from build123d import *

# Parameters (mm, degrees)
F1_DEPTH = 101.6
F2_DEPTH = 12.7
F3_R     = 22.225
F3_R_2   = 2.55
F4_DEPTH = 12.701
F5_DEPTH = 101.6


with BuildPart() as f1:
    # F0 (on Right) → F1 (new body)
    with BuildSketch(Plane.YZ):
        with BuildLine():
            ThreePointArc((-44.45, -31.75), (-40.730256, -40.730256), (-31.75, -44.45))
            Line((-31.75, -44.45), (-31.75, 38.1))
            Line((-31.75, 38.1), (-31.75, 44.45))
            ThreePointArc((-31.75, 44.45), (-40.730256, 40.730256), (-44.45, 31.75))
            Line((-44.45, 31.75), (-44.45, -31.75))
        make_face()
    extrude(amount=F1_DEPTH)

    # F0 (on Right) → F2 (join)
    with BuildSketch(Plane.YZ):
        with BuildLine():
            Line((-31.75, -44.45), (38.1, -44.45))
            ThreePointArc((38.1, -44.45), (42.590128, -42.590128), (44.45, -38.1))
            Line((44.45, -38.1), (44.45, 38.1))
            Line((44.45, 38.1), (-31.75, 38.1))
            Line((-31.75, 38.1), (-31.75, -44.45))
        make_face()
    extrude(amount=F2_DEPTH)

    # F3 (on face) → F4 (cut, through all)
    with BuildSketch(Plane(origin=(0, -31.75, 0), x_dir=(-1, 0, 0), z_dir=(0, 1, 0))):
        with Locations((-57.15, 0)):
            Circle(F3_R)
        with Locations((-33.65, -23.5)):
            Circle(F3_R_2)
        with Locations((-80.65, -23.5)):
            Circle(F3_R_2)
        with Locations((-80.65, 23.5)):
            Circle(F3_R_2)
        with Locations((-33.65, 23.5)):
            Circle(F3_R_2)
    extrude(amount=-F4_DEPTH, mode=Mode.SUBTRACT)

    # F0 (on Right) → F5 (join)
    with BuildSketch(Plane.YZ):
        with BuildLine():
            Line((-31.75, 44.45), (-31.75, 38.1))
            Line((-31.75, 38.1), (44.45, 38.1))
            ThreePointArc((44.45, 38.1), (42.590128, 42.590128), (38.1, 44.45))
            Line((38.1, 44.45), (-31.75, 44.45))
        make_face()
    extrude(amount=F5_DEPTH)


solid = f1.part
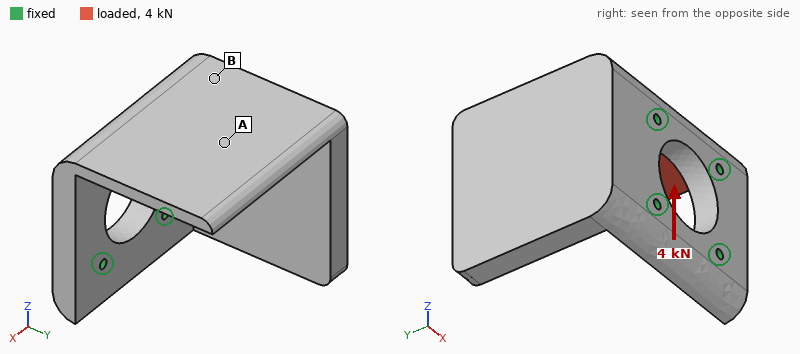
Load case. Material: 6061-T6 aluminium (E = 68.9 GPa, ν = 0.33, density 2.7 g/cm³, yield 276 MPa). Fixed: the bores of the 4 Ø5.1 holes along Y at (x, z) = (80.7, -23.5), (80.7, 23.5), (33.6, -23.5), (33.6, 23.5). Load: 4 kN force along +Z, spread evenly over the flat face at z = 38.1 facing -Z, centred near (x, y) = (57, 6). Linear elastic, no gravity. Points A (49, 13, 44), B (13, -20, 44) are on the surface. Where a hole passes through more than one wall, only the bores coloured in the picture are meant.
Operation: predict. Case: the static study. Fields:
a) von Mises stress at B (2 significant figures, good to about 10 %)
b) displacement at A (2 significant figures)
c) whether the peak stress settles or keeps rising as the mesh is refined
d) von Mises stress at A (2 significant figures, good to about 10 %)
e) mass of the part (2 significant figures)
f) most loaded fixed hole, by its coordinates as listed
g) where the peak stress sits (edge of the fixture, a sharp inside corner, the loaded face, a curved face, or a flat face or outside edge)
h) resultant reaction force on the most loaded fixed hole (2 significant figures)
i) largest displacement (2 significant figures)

20 MPa
0.30 mm
keeps rising
57 MPa
580 g
(33.6, 23.5)
edge of the fixture
3.0 kN
1.1 mm
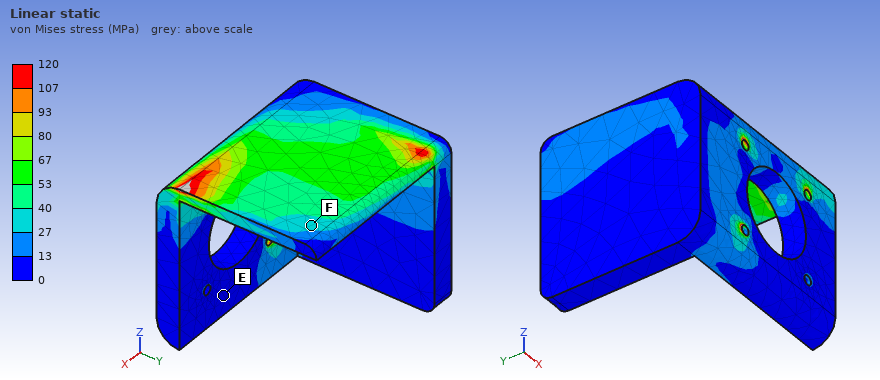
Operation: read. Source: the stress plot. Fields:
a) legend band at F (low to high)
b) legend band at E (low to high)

27 to 40 MPa
0 to 13 MPa
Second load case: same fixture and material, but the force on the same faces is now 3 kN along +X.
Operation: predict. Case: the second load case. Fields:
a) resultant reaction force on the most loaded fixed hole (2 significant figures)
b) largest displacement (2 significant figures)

2.9 kN
0.11 mm
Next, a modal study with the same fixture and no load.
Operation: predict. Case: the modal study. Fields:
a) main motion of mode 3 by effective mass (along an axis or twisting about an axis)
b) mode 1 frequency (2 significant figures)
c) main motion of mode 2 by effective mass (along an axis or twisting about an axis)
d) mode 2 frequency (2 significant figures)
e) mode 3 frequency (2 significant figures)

along Z
1300 Hz
along X
1700 Hz
2100 Hz
